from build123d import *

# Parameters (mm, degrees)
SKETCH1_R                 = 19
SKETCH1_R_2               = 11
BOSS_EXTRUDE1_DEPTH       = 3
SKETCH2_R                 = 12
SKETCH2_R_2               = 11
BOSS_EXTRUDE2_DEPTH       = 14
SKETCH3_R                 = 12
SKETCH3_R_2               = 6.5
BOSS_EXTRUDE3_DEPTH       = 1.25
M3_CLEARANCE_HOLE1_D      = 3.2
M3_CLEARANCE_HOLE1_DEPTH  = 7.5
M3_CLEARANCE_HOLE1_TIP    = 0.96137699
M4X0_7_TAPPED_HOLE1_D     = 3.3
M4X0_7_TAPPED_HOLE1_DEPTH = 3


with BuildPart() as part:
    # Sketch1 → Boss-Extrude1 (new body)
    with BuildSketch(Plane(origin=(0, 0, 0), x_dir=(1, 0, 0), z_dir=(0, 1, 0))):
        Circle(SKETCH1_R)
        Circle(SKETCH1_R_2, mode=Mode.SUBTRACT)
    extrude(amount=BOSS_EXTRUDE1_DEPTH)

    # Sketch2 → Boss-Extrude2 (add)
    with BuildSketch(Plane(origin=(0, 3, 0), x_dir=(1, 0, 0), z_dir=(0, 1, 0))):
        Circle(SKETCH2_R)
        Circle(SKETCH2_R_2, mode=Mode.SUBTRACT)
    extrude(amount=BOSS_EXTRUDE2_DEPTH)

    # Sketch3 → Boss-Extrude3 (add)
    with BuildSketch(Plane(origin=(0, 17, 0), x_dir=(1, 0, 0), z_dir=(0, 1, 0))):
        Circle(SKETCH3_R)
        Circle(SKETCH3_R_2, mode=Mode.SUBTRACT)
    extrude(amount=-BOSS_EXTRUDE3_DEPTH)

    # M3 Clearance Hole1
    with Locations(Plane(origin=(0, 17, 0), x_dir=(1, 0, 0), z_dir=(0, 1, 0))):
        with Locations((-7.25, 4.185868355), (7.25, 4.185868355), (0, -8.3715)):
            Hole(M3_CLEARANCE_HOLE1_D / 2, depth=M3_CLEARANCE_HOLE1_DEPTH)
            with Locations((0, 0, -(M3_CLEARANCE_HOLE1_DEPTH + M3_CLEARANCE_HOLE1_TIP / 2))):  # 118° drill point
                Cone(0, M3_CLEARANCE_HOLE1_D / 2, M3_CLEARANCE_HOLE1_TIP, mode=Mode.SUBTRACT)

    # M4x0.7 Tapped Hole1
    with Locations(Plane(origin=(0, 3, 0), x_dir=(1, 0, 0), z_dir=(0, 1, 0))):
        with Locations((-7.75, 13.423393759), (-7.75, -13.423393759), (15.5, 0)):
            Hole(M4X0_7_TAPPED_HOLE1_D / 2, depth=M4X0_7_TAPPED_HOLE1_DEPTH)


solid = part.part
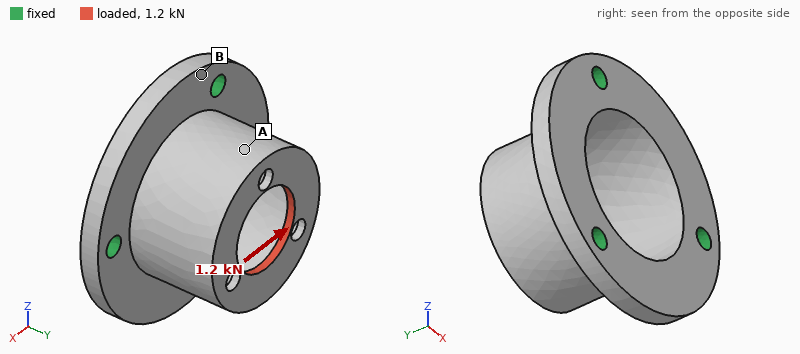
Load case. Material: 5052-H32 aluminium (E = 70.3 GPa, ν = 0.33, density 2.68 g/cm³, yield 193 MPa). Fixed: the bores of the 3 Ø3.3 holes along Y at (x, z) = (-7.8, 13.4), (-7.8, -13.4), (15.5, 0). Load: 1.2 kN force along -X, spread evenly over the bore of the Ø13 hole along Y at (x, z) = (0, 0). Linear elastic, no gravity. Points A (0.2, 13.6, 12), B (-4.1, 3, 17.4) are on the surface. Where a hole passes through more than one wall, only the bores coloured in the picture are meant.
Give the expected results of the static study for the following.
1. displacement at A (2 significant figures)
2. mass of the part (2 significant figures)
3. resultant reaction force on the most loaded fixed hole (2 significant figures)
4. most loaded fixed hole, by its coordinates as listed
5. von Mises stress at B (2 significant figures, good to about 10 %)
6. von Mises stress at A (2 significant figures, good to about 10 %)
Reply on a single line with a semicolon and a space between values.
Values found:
30 µm; 9.3 g; 920 N; (15.5, 0); 16 MPa; 59 MPa
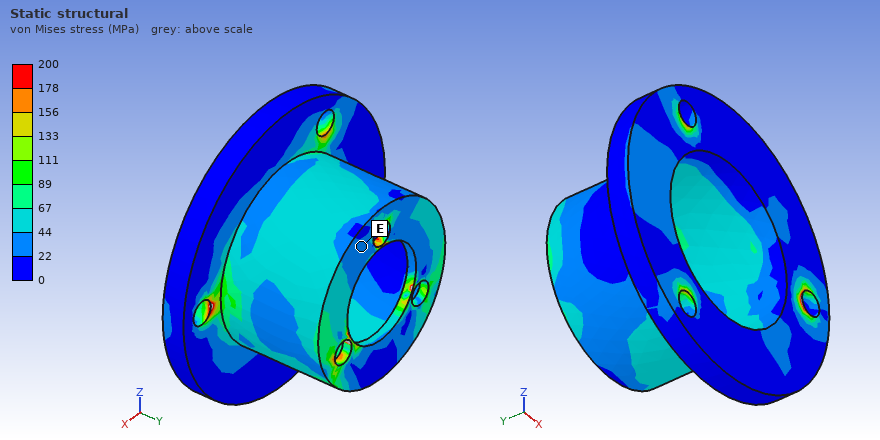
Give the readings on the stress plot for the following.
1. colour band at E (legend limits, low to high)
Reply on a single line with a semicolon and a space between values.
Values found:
22 to 44 MPa
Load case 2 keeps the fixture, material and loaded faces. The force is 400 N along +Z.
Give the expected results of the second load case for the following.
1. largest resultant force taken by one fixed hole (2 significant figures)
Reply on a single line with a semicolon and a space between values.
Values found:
270 N
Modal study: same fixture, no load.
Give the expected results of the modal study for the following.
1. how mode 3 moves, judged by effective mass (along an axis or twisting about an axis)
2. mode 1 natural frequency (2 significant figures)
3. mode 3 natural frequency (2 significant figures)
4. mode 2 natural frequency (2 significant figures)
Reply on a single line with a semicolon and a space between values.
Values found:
along Y; 15 kHz; 19 kHz; 15 kHz
